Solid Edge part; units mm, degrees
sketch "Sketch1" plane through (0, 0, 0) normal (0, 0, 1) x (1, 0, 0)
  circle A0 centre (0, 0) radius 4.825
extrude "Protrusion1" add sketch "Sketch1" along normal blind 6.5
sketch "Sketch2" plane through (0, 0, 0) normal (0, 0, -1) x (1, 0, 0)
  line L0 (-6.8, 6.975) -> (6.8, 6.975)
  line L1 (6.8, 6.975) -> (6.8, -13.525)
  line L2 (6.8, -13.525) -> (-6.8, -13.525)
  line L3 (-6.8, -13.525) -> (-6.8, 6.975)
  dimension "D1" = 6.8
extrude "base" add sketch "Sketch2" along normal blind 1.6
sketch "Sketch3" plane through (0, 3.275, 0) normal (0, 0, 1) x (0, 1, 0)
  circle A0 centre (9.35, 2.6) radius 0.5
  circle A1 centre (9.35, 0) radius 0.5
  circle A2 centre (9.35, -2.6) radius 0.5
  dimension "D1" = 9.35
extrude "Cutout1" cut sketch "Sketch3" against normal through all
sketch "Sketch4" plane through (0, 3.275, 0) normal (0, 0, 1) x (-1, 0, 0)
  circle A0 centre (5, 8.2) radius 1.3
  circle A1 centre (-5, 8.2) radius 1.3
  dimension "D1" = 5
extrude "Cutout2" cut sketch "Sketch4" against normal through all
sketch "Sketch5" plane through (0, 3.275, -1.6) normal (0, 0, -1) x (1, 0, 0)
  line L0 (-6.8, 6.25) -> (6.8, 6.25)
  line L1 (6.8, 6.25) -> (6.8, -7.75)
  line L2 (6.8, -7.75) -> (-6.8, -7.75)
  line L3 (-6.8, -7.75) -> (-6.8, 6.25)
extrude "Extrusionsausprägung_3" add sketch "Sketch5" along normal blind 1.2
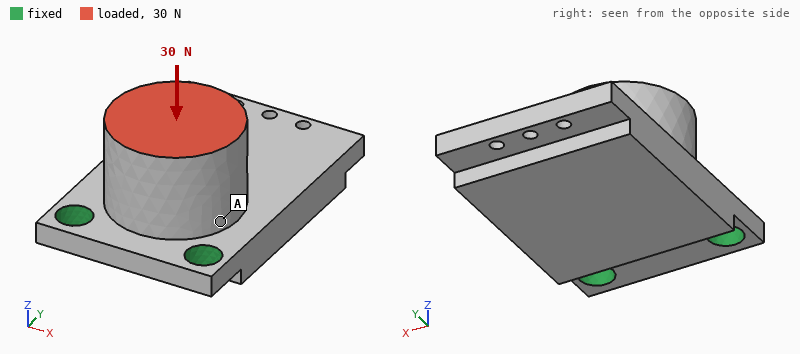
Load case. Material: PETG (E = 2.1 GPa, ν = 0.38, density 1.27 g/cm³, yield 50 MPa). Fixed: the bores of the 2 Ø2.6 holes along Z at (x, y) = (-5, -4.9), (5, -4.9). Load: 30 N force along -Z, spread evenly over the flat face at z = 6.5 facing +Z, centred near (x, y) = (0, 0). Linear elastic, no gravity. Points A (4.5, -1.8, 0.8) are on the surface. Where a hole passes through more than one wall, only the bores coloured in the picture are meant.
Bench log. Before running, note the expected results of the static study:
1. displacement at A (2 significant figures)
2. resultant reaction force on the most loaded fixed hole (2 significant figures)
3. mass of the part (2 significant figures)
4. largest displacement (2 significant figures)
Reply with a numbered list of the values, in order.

1. 0.041 mm
2. 15 N
3. 1.4 g
4. 0.27 mm
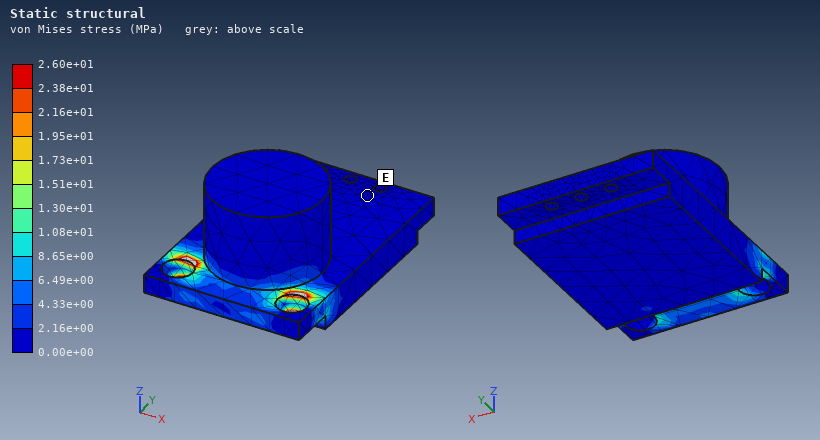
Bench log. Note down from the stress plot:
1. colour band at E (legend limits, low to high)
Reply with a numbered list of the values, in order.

1. 0.00e+00 to 2.16e+00 MPa
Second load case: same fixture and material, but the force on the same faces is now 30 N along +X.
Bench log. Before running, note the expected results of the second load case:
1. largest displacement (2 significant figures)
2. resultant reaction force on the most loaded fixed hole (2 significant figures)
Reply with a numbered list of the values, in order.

1. 39 µm
2. 32 N
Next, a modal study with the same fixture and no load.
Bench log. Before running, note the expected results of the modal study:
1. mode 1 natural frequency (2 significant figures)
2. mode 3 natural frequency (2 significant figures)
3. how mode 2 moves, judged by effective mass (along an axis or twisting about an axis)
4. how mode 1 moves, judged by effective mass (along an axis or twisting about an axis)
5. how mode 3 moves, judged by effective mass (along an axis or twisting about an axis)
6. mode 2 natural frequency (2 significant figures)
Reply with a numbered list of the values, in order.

1. 1400 Hz
2. 6600 Hz
3. along X
4. along Z
5. along X
6. 6000 Hz
